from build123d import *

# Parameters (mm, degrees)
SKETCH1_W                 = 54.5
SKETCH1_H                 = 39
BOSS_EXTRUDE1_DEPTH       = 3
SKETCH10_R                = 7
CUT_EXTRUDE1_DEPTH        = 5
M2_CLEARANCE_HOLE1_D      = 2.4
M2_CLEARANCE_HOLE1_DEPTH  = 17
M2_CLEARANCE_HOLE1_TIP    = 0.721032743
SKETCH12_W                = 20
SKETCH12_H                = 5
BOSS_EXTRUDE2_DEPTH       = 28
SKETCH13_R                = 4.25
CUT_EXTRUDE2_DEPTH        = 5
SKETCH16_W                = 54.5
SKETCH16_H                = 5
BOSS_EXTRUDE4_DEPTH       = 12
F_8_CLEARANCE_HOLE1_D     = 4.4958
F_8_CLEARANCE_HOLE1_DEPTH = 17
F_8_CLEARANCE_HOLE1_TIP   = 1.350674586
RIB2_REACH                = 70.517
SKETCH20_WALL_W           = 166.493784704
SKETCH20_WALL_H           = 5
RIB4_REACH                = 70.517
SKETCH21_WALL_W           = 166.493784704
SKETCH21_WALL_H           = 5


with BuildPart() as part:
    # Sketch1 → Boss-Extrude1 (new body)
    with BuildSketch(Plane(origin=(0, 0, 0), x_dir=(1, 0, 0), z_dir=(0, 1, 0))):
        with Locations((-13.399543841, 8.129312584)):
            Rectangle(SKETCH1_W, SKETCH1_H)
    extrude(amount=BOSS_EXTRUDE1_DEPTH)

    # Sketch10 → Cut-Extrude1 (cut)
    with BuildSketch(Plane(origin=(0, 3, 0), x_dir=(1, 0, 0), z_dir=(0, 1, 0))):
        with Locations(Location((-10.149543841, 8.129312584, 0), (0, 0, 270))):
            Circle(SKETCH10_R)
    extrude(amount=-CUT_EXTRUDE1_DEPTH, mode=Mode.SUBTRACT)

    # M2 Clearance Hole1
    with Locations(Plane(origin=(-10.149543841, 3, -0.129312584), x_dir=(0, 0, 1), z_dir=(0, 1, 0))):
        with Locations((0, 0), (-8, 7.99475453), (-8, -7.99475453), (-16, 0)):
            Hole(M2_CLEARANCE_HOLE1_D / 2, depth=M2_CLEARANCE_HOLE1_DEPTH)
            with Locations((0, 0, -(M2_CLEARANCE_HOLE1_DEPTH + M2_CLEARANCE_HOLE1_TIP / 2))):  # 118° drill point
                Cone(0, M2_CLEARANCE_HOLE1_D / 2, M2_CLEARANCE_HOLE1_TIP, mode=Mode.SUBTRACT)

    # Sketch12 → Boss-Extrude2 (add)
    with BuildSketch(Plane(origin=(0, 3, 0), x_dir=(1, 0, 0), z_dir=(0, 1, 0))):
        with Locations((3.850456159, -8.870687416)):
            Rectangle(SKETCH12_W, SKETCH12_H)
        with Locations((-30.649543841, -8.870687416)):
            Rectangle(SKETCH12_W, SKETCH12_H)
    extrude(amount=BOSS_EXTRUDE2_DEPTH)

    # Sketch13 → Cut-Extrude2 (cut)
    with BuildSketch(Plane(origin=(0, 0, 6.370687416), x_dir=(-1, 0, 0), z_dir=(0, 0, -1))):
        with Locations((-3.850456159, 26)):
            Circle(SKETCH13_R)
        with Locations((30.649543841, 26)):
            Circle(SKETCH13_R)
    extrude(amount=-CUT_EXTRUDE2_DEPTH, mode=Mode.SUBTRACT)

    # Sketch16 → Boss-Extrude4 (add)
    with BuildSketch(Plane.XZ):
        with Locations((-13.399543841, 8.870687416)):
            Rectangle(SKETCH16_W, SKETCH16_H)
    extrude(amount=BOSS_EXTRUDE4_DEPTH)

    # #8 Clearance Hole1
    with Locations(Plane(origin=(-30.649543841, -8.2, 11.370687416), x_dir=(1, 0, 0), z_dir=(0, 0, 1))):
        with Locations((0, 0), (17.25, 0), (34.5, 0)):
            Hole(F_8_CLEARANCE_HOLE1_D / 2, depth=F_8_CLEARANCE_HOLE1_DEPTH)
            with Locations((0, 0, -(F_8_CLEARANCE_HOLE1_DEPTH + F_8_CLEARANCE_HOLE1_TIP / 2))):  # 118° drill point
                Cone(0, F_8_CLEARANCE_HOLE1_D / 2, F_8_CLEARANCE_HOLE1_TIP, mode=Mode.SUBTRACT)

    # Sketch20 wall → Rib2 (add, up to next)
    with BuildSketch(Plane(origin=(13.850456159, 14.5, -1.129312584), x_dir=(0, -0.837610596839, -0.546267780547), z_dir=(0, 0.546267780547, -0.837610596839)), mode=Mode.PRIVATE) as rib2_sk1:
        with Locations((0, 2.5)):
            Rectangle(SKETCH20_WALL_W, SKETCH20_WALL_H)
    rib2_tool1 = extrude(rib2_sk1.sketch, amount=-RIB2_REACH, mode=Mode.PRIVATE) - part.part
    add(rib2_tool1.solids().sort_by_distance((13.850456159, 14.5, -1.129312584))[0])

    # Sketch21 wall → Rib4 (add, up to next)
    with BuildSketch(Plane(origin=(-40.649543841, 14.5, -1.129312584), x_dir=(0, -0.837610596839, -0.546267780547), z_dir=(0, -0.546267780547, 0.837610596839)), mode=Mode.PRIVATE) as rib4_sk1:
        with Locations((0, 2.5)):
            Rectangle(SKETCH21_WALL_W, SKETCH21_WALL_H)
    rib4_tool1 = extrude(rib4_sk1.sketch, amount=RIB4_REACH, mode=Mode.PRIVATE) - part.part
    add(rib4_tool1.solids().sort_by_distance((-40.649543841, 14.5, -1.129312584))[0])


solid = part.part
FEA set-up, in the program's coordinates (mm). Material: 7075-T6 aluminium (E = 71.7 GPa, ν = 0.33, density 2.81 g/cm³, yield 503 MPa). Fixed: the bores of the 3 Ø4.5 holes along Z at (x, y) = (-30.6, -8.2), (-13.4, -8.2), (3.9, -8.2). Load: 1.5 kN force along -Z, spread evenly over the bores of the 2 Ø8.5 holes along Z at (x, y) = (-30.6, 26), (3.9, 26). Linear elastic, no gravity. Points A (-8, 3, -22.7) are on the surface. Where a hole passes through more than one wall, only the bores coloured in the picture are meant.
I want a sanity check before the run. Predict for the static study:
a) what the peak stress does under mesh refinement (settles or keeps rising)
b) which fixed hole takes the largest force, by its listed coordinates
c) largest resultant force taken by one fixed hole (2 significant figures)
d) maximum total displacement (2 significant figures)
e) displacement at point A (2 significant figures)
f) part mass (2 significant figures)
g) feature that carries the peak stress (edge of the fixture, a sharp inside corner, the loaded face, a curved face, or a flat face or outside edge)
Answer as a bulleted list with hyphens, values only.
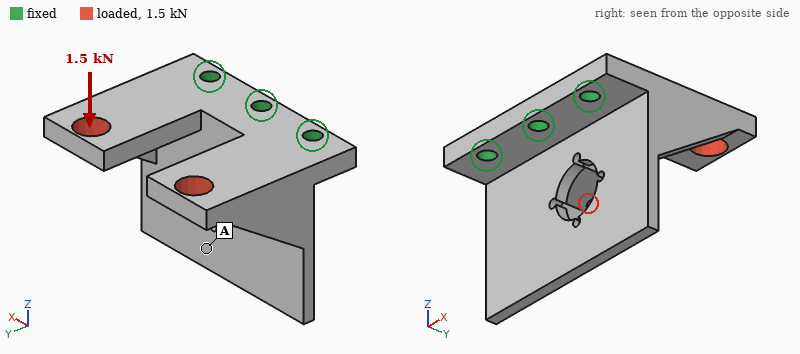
- keeps rising
- (-13.4, -8.2)
- 850 N
- 0.53 mm
- 0.41 mm
- 44 g
- edge of the fixture
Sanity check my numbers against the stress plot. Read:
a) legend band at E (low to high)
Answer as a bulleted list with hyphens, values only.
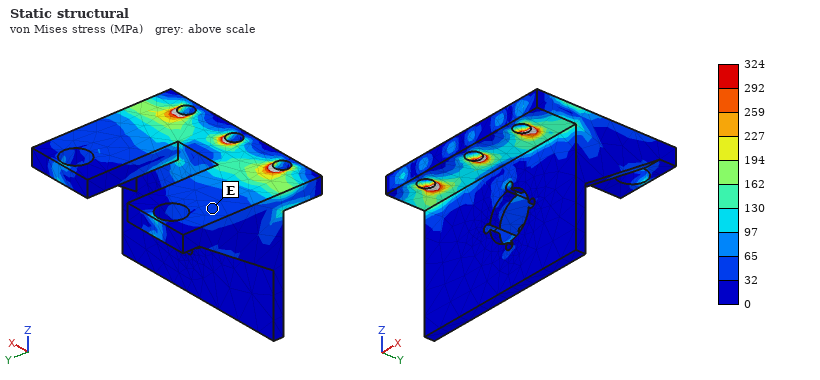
- 32 to 65 MPa
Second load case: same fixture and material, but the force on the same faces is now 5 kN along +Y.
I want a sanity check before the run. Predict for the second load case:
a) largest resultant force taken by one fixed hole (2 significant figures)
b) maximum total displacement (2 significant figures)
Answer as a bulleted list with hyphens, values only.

- 2.2 kN
- 38 µm
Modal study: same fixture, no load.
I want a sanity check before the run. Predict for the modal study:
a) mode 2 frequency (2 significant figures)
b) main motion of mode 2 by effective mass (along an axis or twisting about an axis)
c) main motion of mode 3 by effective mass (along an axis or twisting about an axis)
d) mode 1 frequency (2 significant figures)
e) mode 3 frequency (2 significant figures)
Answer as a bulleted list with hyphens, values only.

- 2900 Hz
- twisting about Y
- along Z
- 2100 Hz
- 4500 Hz
